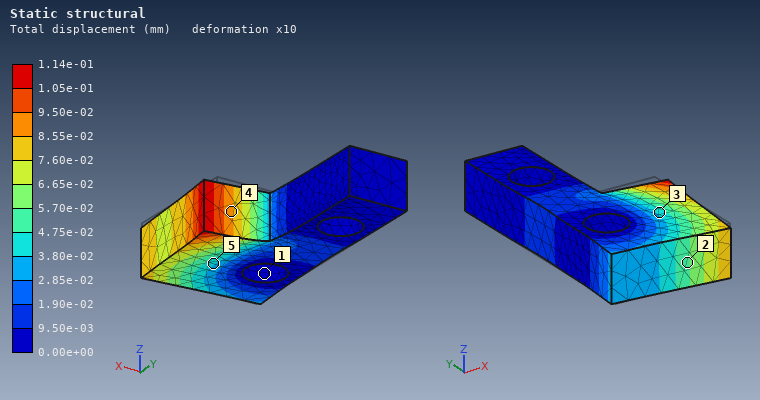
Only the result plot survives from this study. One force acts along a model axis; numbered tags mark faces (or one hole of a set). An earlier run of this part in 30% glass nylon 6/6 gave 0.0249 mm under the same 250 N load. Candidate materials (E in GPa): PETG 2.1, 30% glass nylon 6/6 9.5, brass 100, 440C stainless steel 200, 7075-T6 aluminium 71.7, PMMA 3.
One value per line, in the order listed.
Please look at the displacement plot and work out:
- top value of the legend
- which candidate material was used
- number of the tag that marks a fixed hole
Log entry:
1.14e-01 mm
PETG
1
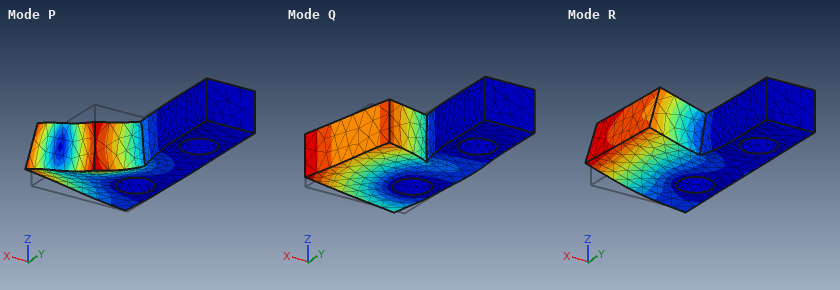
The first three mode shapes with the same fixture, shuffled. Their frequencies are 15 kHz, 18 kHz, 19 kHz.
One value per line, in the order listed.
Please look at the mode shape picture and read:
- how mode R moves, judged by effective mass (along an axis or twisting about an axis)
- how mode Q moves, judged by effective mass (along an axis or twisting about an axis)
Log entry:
along Z
along Y
